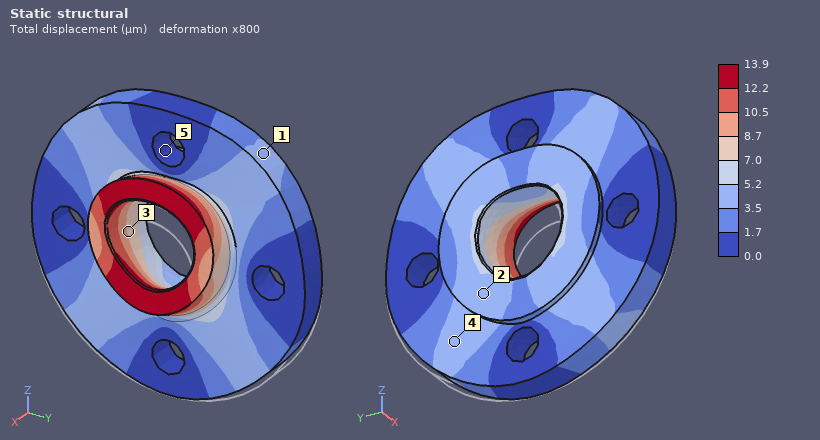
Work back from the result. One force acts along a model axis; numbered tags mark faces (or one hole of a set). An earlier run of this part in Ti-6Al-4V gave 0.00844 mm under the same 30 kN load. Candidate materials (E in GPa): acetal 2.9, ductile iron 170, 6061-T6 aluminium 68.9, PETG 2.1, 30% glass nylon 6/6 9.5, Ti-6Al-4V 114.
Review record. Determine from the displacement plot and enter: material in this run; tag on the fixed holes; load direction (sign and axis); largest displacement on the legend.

6061-T6 aluminium
5
+Z
13.9 µm
